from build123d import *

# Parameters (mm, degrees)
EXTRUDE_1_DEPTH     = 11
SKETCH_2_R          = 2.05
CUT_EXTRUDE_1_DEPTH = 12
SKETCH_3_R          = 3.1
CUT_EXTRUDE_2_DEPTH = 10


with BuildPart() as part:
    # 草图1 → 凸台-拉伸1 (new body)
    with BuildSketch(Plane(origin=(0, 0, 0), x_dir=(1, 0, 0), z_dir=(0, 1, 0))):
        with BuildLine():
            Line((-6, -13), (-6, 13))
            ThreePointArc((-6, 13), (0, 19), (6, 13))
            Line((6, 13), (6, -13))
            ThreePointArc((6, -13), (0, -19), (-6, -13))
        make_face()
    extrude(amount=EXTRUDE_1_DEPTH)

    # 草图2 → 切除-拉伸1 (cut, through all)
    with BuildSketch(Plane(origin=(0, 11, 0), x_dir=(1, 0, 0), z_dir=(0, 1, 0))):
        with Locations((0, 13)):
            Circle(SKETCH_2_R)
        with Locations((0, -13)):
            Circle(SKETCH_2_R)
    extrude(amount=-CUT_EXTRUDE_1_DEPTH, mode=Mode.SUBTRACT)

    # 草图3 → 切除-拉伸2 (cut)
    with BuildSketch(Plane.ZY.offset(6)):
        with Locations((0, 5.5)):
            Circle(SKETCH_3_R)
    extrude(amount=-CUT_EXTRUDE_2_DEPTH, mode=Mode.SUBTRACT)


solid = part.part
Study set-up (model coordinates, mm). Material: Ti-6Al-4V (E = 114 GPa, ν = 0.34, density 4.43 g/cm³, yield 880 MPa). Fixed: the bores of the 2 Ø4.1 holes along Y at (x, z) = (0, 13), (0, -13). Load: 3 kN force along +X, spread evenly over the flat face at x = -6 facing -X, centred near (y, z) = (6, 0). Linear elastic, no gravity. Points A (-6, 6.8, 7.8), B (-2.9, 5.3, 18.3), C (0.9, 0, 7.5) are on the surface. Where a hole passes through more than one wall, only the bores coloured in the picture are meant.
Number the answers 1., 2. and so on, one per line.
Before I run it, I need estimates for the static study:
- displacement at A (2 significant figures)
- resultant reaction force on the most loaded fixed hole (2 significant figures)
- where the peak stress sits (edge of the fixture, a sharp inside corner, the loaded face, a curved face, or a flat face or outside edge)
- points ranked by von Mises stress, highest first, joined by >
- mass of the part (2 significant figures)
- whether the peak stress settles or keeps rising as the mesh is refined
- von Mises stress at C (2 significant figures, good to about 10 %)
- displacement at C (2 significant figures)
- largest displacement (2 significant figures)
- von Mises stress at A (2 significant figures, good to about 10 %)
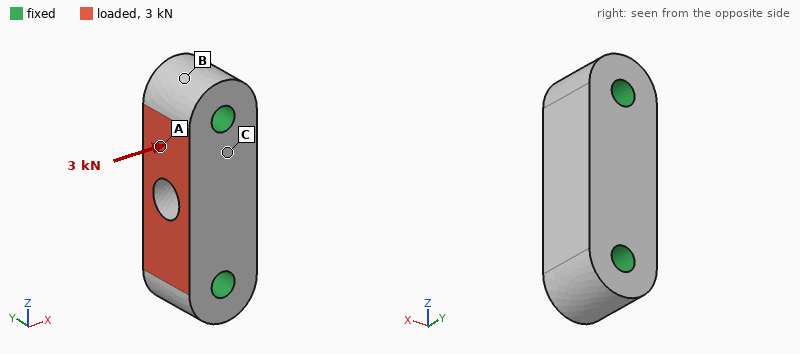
1. 2.4 µm
2. 1.5 kN
3. edge of the fixture
4. C > A > B
5. 18 g
6. keeps rising
7. 18 MPa
8. 1.7 µm
9. 3.8 µm
10. 9.6 MPa
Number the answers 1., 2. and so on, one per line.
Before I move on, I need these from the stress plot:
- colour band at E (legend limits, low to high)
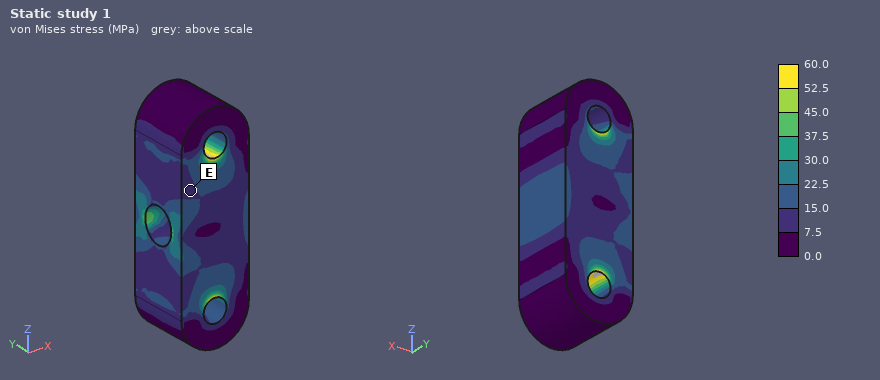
1. 7.5 to 15.0 MPa
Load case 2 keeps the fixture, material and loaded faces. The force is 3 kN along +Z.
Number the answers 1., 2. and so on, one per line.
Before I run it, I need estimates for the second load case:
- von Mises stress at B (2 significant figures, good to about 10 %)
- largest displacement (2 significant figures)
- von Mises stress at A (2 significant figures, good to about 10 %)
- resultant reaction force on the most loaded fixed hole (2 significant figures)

1. 5.3 MPa
2. 2.3 µm
3. 22 MPa
4. 1.6 kN
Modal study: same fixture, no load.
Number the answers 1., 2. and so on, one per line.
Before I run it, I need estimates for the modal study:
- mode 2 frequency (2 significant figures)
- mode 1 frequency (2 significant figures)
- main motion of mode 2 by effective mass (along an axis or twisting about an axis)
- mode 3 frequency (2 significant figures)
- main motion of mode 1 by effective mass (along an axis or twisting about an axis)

1. 53 kHz
2. 46 kHz
3. along Y
4. 59 kHz
5. along X
